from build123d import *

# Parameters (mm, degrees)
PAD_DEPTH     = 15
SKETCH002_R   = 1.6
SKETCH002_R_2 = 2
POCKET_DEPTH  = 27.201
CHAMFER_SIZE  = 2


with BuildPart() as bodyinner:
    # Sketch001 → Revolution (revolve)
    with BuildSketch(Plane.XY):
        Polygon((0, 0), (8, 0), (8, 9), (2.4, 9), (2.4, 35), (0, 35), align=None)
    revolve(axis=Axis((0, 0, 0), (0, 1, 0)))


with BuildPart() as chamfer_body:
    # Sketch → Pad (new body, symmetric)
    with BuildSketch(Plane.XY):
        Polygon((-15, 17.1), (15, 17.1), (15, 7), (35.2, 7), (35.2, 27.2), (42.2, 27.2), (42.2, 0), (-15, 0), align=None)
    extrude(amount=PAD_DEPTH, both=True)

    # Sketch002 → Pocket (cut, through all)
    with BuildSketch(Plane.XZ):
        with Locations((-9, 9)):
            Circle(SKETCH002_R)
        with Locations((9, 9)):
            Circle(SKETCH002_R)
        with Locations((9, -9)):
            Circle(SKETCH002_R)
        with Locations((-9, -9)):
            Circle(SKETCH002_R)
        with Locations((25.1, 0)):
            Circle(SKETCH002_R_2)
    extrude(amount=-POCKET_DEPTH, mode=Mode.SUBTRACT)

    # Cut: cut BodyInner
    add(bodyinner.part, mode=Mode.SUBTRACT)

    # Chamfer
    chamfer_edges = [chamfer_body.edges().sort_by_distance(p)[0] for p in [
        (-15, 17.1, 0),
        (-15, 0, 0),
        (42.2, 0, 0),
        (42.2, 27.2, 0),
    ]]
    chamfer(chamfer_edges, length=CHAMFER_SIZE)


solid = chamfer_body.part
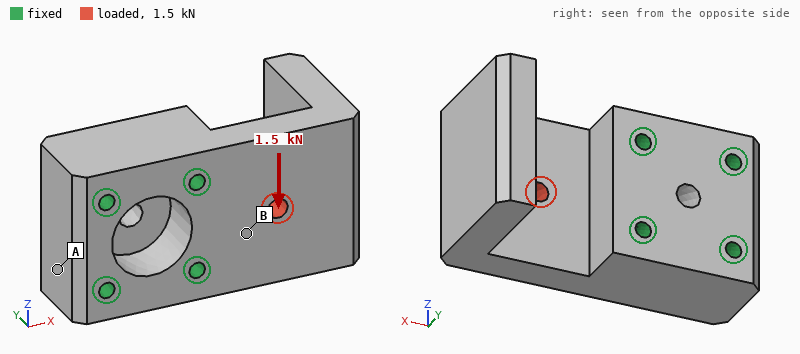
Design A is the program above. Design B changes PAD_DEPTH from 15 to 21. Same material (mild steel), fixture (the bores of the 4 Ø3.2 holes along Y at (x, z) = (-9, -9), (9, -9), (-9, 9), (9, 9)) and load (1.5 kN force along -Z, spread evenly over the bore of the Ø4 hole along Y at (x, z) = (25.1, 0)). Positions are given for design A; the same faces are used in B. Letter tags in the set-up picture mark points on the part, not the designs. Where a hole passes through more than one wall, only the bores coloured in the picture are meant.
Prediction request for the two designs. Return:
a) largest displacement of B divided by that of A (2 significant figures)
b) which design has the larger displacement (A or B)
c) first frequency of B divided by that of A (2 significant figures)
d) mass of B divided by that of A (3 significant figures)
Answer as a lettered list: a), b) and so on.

a) 0.66
b) A
c) 1.0
d) 1.45
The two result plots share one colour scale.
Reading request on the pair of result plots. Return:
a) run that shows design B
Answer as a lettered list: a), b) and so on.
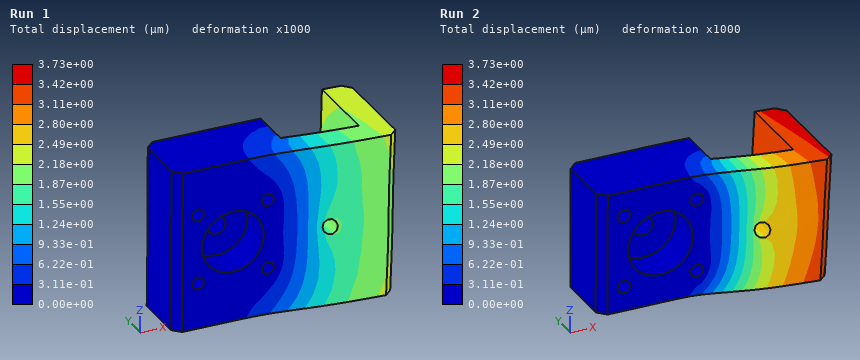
a) Run 1
